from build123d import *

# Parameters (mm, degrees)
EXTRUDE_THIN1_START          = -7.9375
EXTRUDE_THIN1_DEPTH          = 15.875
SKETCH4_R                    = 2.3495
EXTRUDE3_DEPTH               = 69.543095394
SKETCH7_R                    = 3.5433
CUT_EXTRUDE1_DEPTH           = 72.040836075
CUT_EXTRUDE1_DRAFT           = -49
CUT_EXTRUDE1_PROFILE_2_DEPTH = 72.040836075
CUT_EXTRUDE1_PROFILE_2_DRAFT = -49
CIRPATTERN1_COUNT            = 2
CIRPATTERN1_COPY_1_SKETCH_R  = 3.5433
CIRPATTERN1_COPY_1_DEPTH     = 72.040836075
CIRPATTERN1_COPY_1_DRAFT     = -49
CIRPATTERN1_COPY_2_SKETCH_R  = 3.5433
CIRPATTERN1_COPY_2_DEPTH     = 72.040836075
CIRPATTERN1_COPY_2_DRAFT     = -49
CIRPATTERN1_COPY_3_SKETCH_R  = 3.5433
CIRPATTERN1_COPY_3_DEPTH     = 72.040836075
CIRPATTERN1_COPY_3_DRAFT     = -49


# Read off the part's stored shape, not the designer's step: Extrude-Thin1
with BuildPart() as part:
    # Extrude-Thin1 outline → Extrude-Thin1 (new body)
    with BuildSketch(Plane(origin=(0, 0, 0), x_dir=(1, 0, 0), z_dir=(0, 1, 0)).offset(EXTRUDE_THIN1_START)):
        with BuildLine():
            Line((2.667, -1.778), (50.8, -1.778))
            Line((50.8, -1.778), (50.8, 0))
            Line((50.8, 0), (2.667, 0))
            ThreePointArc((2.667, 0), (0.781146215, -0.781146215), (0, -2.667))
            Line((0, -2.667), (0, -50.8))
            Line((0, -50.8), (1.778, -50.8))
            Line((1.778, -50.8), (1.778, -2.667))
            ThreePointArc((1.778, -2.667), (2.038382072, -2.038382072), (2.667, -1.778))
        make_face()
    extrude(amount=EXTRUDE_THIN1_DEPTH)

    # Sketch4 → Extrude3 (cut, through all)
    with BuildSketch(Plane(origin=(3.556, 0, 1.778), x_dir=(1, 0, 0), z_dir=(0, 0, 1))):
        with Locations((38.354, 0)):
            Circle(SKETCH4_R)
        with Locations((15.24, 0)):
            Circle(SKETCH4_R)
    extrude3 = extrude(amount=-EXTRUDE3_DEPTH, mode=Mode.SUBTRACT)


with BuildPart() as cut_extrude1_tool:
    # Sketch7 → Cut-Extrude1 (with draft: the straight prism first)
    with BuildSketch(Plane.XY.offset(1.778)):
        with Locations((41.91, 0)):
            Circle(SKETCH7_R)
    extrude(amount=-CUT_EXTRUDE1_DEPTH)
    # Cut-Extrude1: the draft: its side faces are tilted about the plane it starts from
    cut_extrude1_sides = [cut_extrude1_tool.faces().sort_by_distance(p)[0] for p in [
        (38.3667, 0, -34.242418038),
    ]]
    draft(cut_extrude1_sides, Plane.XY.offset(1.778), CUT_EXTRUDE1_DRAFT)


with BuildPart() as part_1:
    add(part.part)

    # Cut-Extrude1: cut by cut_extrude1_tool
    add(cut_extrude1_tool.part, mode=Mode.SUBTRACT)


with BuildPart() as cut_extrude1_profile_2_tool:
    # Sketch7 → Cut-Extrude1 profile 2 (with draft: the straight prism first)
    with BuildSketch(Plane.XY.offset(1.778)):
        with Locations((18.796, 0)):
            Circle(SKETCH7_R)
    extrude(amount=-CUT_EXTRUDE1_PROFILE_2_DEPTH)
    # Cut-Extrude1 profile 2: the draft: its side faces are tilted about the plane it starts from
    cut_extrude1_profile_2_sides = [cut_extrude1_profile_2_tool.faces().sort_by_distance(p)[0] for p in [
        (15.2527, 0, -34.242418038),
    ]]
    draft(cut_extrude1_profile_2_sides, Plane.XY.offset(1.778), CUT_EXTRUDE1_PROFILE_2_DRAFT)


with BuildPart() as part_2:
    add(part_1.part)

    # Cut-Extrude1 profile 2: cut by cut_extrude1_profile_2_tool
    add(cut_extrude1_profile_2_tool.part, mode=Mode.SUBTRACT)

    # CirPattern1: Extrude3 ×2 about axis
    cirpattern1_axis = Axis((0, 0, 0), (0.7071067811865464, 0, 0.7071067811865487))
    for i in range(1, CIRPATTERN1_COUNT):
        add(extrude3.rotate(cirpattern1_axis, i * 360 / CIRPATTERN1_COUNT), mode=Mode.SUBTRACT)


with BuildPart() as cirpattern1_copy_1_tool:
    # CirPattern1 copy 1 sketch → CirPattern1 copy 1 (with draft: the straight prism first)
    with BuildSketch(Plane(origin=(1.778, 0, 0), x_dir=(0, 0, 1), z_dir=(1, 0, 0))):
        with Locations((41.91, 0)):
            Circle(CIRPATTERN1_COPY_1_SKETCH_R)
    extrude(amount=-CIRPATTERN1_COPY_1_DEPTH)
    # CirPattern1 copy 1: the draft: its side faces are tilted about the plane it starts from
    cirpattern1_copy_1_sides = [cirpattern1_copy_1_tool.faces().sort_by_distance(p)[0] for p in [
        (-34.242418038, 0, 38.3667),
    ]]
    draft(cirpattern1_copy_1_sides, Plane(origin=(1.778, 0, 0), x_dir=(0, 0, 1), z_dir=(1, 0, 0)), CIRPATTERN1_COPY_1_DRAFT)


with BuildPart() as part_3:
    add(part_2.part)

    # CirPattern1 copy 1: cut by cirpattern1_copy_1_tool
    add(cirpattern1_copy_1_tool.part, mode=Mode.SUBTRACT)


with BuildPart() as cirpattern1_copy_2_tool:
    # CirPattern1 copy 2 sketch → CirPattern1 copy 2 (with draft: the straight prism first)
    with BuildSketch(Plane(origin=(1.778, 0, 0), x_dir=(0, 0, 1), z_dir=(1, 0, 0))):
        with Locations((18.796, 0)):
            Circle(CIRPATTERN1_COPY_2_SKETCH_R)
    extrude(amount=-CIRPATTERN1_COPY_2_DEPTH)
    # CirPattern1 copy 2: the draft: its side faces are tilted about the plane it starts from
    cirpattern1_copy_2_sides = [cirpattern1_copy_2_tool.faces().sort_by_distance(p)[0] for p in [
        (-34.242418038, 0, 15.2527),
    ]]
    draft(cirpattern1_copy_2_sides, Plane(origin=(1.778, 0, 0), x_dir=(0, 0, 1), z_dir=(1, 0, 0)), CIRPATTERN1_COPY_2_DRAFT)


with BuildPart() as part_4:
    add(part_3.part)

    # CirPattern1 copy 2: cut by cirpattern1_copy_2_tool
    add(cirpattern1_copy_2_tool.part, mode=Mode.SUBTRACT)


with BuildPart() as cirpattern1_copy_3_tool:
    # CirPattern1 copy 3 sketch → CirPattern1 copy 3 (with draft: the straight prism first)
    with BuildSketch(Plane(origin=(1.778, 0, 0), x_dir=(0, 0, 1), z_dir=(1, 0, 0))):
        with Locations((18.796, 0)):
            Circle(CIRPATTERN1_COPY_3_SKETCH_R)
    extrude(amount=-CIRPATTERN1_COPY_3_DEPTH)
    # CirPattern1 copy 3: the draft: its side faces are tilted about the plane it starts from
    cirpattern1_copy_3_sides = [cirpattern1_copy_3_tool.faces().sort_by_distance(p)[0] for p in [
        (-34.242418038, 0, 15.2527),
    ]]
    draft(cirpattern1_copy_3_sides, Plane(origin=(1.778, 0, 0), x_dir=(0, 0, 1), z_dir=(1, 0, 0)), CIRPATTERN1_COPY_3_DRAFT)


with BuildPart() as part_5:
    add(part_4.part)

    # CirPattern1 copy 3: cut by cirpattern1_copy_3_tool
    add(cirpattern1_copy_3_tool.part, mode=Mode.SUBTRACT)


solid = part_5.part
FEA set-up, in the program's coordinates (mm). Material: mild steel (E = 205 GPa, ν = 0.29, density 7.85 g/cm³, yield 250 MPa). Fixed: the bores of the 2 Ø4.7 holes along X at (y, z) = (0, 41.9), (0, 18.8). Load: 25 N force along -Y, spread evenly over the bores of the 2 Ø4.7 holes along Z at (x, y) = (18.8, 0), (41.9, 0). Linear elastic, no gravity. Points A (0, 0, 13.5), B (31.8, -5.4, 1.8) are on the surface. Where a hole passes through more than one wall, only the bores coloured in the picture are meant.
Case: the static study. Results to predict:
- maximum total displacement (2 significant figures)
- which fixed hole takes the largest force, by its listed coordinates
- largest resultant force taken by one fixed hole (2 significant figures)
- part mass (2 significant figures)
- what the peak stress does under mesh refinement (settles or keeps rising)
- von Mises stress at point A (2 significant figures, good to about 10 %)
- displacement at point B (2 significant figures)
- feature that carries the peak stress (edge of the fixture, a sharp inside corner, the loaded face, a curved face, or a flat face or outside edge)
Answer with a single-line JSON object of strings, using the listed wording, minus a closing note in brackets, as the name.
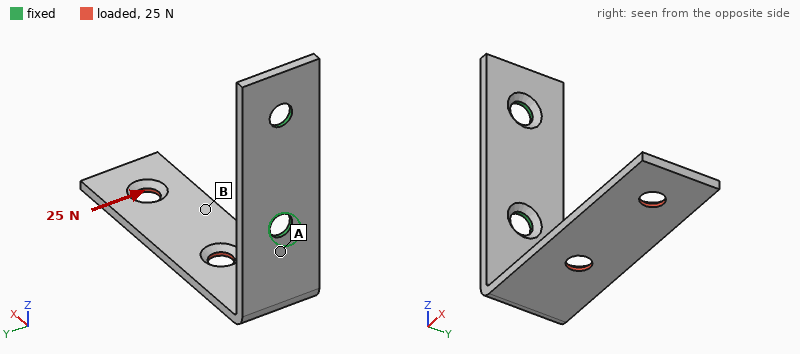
{"maximum total displacement": "0.28 mm", "which fixed hole takes the largest force, by its listed coordinates": "(0, 18.8)", "largest resultant force taken by one fixed hole": "29 N", "part mass": "21 g", "what the peak stress does under mesh refinement": "keeps rising", "von Mises stress at point A": "77 MPa", "displacement at point B": "0.17 mm", "feature that carries the peak stress": "edge of the fixture"}
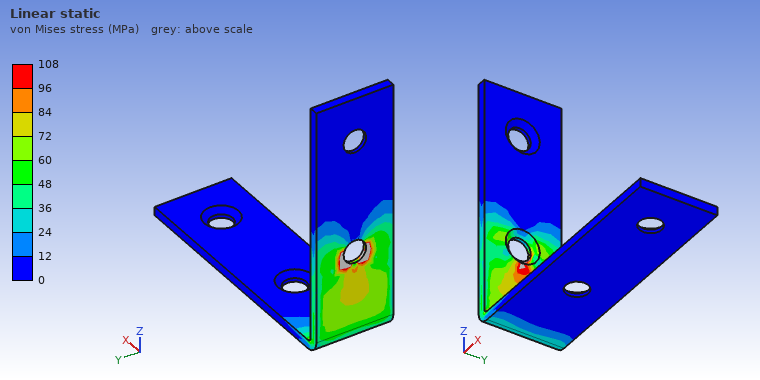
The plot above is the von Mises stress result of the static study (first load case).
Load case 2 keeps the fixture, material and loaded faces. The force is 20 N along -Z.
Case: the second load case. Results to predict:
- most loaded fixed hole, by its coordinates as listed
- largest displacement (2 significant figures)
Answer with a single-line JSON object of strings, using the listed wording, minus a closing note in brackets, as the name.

{"most loaded fixed hole, by its coordinates as listed": "(0, 41.9)", "largest displacement": "0.60 mm"}
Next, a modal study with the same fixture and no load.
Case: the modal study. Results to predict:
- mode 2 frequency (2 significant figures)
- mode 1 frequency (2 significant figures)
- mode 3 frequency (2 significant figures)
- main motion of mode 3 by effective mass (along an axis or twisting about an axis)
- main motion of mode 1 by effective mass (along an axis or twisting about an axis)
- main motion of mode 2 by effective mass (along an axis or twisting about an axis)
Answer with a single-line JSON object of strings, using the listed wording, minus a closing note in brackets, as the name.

{"mode 2 frequency": "620 Hz", "mode 1 frequency": "380 Hz", "mode 3 frequency": "1700 Hz", "main motion of mode 3 by effective mass": "along X", "main motion of mode 1 by effective mass": "along Z", "main motion of mode 2 by effective mass": "along Y"}
